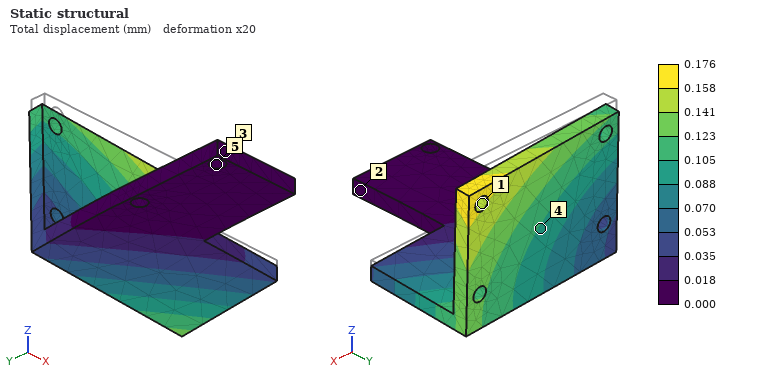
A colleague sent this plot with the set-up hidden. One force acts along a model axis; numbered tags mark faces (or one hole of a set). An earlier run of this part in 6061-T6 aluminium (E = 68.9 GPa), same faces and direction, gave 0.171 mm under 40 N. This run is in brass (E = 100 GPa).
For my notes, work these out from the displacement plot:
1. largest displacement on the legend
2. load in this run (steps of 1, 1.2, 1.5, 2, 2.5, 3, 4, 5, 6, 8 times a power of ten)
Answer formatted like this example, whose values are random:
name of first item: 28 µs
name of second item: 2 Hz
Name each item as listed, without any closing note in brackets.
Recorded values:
largest displacement on the legend: 0.176 mm
load in this run: 60 N
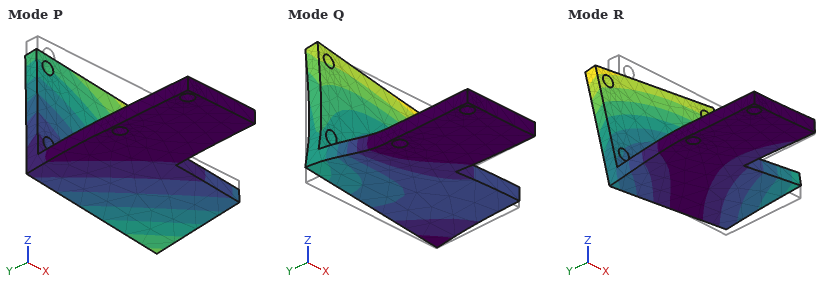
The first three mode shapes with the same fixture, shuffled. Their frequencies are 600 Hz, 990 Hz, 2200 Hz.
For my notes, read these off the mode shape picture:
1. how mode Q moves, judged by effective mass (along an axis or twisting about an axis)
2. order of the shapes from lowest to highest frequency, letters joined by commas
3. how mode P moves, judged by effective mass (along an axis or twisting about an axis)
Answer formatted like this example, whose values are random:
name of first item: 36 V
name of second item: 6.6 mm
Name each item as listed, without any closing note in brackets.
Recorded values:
how mode Q moves, judged by effective mass: along Z
order of the shapes from lowest to highest frequency, letters joined by commas: P, R, Q
how mode P moves, judged by effective mass: along Z
